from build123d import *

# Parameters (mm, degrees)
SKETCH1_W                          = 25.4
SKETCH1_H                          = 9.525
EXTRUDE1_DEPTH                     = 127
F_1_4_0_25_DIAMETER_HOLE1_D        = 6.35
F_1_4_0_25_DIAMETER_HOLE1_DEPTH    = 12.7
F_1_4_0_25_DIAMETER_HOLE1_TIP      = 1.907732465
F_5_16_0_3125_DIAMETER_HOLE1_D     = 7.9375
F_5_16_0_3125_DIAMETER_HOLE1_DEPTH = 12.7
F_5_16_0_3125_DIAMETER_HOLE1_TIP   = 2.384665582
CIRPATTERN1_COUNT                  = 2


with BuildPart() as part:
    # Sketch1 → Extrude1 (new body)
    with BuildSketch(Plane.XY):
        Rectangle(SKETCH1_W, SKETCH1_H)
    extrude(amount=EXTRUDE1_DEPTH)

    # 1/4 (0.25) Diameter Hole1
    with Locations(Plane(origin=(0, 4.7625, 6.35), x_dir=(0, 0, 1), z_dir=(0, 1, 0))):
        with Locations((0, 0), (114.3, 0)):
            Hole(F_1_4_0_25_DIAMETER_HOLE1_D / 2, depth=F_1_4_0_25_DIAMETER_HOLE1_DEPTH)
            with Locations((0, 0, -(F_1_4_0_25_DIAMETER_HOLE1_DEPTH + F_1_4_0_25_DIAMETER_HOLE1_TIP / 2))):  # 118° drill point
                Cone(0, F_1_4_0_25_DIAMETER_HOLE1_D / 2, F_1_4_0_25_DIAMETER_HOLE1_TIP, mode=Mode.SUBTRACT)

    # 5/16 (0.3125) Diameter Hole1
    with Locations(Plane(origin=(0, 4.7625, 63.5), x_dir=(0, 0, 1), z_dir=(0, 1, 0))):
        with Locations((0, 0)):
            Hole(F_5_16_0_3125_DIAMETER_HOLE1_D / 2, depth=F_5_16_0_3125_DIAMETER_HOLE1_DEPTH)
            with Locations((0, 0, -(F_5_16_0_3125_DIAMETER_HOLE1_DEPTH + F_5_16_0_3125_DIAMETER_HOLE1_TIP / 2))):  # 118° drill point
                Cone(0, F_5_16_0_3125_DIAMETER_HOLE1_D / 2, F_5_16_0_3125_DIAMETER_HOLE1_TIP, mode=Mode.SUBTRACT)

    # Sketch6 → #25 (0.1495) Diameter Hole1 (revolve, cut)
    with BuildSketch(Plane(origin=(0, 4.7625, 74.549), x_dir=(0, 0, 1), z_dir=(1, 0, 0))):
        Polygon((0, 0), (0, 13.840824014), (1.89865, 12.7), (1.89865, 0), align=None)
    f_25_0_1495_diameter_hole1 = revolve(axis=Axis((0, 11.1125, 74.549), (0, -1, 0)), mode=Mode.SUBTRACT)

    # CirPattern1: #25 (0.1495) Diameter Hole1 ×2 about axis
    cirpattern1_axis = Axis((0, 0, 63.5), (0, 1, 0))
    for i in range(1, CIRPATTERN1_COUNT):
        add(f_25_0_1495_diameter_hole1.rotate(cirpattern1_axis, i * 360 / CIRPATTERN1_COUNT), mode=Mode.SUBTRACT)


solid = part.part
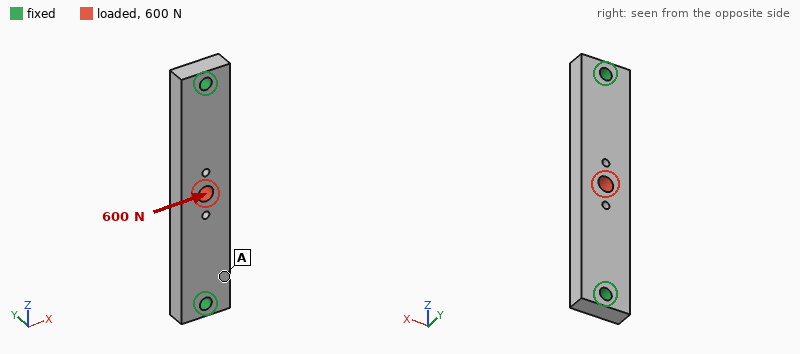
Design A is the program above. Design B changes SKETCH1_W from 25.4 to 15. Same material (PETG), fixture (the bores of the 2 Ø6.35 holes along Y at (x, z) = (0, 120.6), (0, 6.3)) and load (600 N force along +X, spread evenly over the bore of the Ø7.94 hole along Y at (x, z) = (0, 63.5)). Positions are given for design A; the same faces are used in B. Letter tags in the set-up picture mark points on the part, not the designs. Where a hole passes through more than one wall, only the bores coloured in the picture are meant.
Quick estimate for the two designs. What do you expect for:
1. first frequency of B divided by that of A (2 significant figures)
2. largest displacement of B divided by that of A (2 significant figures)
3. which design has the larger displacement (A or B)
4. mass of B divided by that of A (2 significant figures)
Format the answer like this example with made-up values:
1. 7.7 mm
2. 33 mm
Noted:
1. 1.0
2. 2.6
3. B
4. 0.57
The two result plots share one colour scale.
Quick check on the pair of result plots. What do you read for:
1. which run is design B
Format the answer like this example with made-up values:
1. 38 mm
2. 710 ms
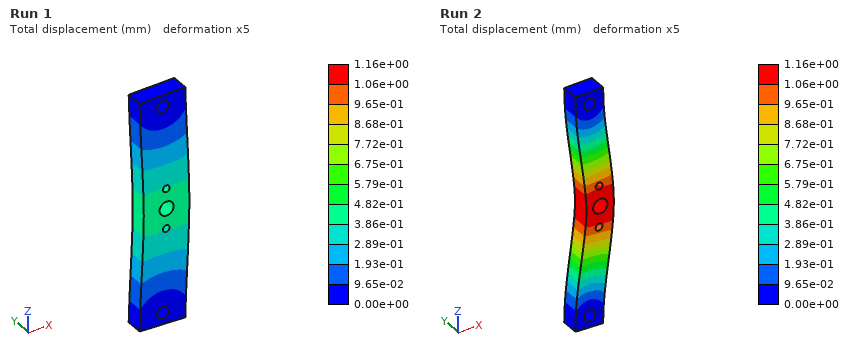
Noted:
1. Run 2
